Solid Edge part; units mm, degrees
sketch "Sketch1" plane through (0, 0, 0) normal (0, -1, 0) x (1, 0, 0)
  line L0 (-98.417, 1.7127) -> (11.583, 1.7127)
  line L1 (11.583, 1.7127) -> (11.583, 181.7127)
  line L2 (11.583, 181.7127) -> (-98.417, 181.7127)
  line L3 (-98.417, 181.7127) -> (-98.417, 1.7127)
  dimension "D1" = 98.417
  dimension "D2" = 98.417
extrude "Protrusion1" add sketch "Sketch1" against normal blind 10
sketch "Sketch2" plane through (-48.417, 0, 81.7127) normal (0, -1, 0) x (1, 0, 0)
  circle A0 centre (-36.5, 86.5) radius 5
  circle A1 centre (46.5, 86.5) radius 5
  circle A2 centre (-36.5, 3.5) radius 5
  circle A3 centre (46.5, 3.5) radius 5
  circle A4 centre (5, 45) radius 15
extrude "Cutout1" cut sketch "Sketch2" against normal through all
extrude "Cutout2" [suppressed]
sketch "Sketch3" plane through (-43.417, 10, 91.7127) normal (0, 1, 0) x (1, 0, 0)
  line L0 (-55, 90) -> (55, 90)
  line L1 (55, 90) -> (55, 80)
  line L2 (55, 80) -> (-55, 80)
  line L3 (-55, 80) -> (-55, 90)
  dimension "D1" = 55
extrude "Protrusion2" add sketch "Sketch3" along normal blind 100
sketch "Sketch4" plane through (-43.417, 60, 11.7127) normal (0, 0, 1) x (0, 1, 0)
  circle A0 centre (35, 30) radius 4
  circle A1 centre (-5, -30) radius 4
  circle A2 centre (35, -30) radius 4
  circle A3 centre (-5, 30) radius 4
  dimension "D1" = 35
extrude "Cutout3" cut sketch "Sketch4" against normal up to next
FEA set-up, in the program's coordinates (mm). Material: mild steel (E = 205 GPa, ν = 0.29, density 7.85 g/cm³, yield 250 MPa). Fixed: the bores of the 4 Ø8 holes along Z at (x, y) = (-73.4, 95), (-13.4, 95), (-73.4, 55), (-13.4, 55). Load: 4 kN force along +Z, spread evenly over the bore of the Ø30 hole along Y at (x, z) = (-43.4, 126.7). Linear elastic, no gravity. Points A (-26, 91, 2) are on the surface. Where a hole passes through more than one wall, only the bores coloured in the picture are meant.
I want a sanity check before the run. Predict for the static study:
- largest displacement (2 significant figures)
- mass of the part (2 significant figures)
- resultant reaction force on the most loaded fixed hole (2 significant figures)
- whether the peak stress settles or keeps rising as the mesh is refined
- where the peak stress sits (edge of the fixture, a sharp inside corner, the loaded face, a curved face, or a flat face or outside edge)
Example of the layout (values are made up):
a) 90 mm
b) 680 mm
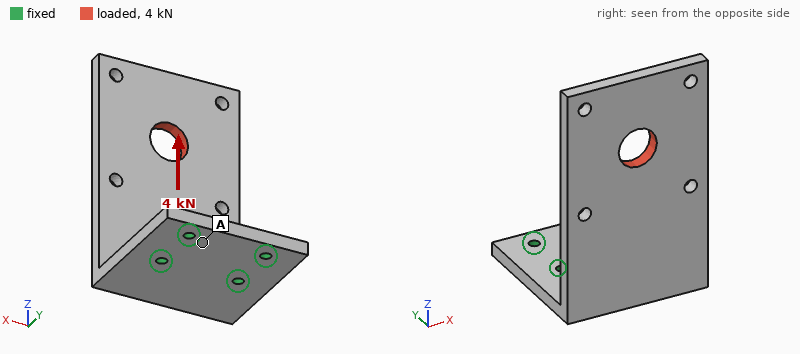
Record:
a) 0.50 mm
b) 2.3 kg
c) 2.9 kN
d) keeps rising
e) edge of the fixture
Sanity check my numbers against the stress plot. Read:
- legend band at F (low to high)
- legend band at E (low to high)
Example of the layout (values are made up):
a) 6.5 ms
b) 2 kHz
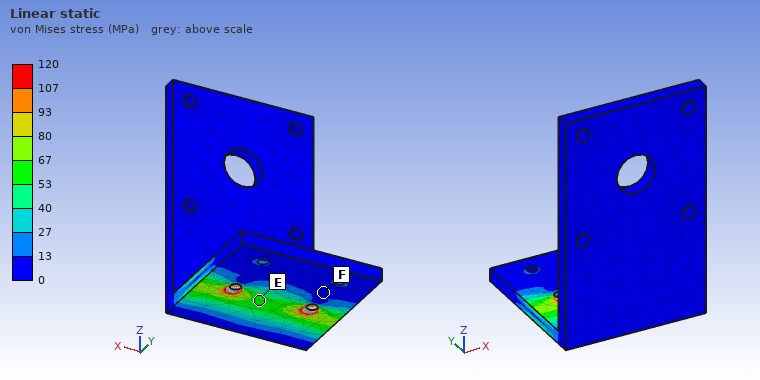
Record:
a) 0 to 13 MPa
b) 53 to 67 MPa
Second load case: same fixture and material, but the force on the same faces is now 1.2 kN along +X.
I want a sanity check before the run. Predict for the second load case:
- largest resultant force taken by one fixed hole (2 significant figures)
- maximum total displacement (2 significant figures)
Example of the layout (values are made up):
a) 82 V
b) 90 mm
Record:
a) 2.5 kN
b) 0.21 mm
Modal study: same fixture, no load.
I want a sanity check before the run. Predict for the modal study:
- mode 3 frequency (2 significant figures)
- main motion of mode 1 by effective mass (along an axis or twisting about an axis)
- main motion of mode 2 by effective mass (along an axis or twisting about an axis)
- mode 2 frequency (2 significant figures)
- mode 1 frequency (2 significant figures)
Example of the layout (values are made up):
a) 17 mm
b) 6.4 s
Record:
a) 910 Hz
b) along Y
c) along X
d) 450 Hz
e) 190 Hz
